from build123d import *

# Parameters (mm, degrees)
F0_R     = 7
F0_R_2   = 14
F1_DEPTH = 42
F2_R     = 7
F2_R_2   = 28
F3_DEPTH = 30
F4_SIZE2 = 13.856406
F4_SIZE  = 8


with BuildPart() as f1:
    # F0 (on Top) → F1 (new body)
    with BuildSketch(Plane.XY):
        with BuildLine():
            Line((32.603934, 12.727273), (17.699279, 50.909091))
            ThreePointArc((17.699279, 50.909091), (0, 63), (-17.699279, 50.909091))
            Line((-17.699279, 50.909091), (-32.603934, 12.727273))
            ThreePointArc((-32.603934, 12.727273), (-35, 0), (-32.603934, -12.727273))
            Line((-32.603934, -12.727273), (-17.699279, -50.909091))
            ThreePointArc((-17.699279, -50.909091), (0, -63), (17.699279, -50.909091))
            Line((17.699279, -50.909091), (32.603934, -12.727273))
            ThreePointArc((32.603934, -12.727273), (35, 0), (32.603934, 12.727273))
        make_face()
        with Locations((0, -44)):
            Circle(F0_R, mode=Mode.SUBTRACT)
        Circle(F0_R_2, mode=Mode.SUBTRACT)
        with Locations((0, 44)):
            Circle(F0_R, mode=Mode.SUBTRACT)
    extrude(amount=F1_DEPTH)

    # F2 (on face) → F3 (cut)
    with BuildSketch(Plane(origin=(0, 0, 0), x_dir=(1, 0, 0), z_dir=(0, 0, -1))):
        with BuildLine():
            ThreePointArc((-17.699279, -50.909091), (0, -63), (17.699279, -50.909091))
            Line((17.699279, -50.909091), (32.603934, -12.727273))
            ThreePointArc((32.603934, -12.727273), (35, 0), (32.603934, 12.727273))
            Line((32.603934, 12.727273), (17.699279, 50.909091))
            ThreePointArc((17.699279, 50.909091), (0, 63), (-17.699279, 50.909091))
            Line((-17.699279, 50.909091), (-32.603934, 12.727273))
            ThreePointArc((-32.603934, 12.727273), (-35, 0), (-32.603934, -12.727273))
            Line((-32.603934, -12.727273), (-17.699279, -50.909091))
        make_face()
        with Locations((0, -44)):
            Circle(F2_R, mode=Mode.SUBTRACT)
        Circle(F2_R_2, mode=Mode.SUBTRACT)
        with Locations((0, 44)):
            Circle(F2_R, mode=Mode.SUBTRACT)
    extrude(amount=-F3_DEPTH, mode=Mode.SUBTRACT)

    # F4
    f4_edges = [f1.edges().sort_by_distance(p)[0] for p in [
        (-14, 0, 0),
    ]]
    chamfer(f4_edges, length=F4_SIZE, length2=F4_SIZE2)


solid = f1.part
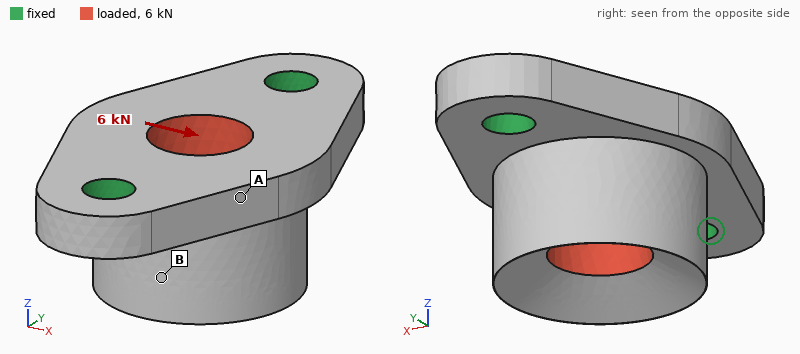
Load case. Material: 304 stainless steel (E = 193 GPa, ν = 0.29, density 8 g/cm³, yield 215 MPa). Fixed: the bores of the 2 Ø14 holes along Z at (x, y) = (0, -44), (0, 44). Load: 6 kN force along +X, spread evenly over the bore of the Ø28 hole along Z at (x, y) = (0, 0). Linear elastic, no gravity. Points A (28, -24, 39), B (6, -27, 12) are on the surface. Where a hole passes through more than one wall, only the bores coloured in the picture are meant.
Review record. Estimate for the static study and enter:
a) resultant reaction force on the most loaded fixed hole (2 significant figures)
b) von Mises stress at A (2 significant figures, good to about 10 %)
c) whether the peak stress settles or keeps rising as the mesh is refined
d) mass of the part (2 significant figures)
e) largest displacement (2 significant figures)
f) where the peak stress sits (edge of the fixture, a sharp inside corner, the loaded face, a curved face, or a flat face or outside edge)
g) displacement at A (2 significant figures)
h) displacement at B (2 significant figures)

3.0 kN
13 MPa
keeps rising
900 g
15 µm
edge of the fixture
7.0 µm
9.1 µm
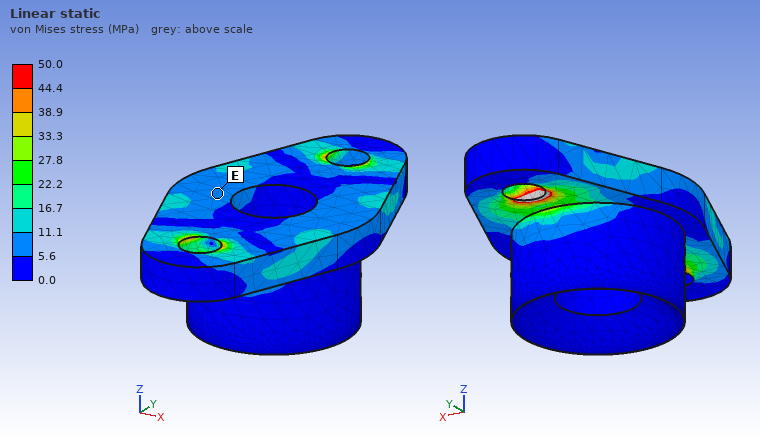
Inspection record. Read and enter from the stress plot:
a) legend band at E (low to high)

5.6 to 11.1 MPa
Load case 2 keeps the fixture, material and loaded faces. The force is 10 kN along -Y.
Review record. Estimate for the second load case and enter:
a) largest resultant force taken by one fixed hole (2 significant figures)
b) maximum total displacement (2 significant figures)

5.2 kN
4.2 µm
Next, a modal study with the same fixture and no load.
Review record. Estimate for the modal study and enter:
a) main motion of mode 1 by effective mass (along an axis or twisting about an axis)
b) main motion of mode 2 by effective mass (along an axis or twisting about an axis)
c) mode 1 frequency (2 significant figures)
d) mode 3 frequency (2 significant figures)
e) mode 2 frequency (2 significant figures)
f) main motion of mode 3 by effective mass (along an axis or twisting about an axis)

along X
along Z
3800 Hz
10 kHz
6800 Hz
along Y
